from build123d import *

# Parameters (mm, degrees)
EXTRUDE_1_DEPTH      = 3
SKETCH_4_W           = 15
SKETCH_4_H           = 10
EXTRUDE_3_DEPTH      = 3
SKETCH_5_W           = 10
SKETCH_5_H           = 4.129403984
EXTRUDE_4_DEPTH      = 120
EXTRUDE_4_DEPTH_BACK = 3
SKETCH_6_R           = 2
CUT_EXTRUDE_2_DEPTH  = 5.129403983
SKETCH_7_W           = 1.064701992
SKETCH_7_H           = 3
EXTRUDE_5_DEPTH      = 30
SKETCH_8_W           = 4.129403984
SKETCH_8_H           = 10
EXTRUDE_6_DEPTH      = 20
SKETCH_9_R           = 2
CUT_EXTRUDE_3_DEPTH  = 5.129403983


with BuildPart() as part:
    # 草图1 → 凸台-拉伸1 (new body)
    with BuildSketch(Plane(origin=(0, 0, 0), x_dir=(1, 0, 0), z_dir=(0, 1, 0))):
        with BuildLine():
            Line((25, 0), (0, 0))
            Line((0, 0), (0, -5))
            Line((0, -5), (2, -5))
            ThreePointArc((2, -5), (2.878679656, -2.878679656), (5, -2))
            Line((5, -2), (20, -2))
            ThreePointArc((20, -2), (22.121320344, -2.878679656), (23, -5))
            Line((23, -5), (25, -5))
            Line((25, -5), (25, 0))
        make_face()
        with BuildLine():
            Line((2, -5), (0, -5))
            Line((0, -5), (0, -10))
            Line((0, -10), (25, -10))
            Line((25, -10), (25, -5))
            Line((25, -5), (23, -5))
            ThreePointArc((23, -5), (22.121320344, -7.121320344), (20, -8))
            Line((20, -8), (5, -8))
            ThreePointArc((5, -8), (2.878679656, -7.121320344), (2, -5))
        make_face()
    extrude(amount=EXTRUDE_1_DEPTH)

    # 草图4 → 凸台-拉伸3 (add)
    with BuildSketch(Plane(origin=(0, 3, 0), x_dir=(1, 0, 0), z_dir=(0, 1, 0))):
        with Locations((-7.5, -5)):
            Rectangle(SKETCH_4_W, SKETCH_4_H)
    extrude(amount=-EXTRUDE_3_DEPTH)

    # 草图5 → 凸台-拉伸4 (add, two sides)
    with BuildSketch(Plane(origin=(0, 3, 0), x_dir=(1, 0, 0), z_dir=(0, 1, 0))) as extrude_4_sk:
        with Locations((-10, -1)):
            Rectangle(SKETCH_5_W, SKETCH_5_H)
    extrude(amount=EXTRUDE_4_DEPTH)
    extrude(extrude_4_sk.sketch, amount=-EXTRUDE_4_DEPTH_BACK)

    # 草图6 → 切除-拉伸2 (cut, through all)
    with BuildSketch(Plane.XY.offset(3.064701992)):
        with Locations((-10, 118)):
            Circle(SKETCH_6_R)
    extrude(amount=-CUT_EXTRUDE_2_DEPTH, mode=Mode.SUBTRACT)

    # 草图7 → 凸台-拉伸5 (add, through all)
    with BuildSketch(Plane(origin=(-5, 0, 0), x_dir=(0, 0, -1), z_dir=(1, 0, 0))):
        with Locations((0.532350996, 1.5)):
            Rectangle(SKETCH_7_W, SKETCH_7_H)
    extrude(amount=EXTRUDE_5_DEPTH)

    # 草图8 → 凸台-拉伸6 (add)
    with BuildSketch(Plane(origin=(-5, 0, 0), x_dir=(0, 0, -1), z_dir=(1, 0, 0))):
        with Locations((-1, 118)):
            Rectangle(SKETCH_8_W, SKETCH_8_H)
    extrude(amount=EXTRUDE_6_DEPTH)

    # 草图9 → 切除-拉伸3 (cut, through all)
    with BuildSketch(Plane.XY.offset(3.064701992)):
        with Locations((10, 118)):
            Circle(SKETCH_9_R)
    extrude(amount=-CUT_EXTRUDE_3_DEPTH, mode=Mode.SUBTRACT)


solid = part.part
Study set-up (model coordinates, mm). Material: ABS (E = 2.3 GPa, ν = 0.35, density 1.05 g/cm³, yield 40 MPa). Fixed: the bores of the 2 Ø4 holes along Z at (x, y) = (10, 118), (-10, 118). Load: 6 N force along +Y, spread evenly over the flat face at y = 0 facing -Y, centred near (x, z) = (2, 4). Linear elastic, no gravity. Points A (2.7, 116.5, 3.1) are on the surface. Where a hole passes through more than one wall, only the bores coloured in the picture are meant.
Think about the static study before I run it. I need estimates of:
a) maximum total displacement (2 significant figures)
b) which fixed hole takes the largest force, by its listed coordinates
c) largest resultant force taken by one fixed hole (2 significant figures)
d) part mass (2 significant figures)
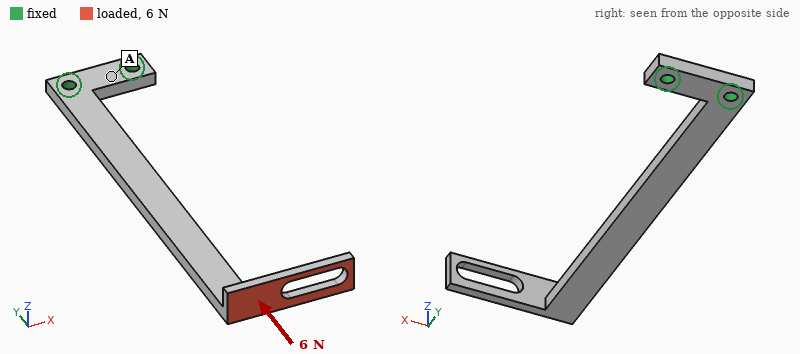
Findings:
1.5 mm
(-10, 118)
4.1 N
7.0 g
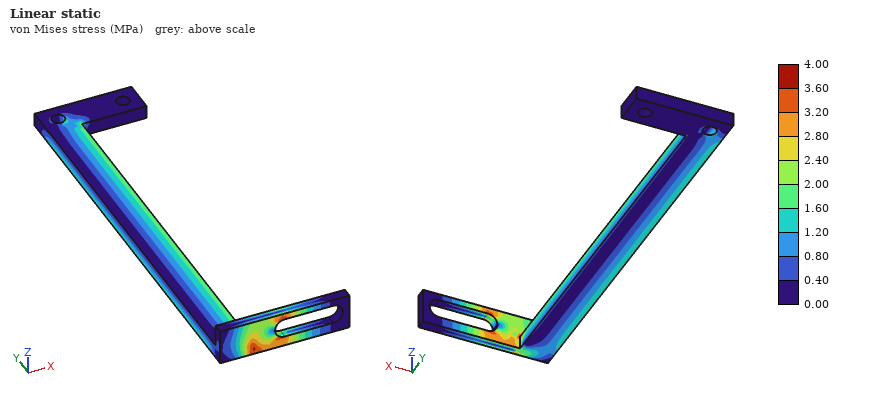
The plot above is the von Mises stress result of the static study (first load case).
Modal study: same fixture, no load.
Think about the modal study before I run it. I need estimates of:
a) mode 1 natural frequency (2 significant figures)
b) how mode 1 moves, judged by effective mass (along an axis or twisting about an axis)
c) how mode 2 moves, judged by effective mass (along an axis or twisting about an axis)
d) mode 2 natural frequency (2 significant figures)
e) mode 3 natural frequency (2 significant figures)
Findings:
56 Hz
along Z
along X
130 Hz
320 Hz
